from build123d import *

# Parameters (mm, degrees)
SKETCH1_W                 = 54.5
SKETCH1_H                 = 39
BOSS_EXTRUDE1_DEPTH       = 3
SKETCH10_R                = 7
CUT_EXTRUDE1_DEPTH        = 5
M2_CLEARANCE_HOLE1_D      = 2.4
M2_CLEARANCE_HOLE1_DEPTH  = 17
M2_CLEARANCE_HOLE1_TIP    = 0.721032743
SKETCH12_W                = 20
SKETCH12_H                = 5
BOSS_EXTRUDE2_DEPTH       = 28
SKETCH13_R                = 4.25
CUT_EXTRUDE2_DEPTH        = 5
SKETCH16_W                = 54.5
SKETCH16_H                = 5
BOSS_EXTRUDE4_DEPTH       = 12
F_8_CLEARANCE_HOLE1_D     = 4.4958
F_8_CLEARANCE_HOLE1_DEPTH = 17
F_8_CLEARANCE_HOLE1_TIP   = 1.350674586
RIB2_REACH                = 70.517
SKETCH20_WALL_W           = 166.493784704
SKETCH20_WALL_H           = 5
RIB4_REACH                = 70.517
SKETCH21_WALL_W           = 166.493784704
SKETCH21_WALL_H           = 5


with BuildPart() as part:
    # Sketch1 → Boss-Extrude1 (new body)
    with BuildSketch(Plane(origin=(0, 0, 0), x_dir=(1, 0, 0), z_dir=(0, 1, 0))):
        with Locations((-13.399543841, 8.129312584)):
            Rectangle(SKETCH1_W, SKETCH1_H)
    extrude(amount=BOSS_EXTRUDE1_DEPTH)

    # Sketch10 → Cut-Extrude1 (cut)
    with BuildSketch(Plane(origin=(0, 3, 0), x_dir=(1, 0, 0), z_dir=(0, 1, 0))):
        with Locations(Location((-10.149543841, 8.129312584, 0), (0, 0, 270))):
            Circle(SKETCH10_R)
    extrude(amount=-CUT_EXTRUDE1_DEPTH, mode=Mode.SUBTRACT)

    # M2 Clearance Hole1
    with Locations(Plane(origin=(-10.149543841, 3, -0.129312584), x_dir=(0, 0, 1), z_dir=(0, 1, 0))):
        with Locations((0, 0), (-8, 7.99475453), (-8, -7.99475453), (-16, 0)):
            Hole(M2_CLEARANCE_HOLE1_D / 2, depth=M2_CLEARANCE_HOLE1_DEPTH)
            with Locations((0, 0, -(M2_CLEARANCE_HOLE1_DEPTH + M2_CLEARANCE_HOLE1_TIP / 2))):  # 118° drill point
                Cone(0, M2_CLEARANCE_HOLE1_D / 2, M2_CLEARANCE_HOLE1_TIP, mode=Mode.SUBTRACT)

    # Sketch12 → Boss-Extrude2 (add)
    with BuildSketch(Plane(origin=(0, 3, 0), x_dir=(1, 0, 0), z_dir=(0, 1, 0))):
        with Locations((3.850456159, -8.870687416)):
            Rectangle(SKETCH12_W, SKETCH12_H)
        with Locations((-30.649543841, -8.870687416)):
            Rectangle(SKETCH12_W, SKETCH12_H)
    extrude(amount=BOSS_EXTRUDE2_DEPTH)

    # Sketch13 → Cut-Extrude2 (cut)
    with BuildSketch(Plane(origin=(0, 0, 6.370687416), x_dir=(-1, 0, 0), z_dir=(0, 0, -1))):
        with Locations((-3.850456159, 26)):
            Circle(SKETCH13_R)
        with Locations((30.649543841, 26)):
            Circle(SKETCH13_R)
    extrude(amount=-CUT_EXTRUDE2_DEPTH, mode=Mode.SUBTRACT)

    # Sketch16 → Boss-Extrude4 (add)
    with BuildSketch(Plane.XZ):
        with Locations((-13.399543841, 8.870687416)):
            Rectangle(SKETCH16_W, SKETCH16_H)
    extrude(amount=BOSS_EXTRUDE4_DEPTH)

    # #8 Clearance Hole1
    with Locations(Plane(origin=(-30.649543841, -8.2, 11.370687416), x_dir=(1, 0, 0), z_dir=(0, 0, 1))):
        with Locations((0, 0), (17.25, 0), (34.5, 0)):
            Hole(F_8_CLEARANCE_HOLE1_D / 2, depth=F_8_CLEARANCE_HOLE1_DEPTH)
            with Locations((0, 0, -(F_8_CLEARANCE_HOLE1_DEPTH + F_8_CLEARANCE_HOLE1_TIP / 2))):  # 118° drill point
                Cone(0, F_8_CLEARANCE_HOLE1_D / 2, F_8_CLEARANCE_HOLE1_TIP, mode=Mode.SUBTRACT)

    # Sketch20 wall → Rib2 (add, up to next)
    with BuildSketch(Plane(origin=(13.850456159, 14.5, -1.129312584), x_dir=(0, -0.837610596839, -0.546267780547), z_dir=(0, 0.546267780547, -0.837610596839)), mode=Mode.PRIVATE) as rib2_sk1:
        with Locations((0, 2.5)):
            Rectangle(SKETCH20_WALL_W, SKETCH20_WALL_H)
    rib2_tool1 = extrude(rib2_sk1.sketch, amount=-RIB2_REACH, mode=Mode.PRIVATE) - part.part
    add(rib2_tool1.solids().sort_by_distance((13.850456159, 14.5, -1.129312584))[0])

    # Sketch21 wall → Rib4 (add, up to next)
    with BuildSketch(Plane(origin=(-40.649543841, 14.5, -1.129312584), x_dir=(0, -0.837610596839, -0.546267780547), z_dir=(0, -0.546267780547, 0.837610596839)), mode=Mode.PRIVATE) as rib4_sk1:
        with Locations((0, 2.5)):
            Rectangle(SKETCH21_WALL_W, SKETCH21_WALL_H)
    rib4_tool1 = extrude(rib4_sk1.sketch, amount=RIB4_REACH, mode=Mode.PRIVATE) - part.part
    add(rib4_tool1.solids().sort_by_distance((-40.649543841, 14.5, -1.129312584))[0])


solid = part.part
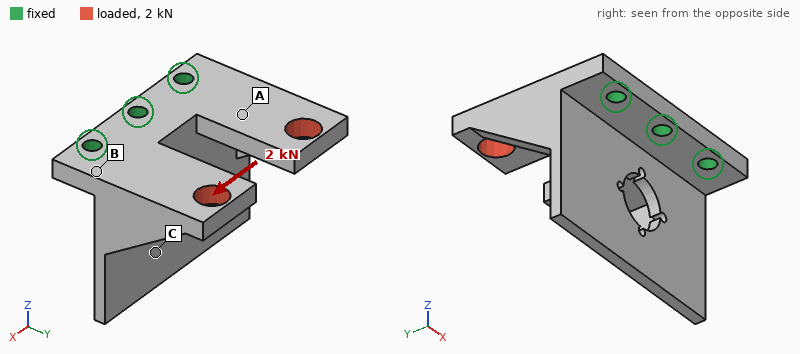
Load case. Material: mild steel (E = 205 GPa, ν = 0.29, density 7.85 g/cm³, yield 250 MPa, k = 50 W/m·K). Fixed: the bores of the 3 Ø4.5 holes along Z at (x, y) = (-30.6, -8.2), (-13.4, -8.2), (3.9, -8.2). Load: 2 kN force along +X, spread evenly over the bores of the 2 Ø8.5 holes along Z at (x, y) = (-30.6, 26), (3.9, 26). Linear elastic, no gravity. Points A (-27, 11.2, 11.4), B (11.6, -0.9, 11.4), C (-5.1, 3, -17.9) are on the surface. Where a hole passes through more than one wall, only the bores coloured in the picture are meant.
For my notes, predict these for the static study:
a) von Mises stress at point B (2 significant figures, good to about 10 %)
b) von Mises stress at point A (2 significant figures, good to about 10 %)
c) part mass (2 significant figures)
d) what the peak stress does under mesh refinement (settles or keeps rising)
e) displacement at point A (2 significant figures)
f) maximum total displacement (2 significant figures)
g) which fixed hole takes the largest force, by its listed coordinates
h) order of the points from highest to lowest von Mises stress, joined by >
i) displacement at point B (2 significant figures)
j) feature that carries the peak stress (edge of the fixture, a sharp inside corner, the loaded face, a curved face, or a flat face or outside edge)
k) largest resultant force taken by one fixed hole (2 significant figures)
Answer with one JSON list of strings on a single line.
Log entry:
["34 MPa", "27 MPa", "120 g", "keeps rising", "9.0 µm", "32 µm", "(-13.4, -8.2)", "B > A > C", "4.8 µm", "edge of the fixture", "2.1 kN"]
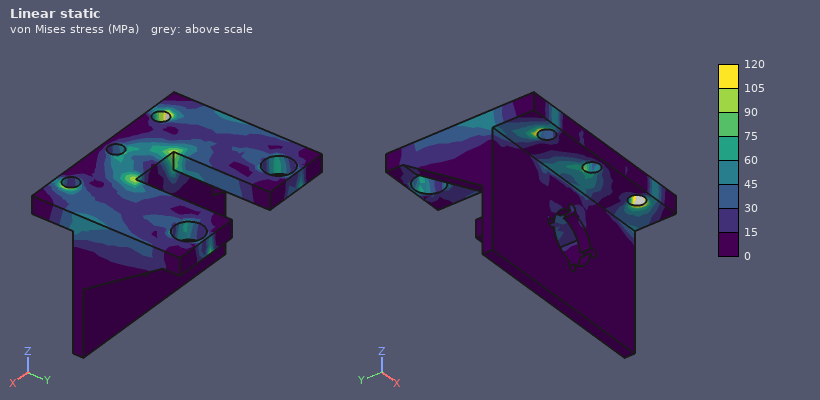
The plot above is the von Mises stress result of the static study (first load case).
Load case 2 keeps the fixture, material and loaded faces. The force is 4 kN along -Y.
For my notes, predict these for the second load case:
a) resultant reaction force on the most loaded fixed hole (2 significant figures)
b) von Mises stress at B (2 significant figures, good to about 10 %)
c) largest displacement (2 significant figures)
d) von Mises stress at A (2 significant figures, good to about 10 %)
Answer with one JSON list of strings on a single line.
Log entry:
["1.8 kN", "16 MPa", "11 µm", "23 MPa"]
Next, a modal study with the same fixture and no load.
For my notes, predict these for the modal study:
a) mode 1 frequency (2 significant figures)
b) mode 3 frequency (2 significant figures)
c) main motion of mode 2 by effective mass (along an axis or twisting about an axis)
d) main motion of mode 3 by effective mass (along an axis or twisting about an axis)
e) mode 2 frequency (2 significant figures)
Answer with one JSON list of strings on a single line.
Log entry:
["2100 Hz", "4600 Hz", "twisting about Y", "along Z", "3000 Hz"]
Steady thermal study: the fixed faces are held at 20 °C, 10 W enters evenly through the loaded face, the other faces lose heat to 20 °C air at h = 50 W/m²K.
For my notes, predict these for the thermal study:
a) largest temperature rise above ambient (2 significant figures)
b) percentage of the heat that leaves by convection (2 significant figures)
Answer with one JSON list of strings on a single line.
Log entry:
["29 K", "36 %"]
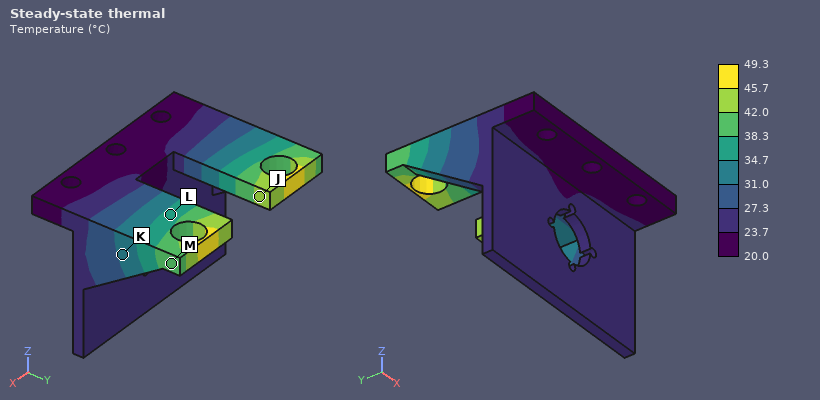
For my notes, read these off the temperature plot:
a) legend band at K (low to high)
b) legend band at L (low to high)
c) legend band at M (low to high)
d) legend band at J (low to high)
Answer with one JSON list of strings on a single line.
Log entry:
["31.0 to 34.7 °C", "34.7 to 38.3 °C", "38.3 to 42.0 °C", "42.0 to 45.7 °C"]
